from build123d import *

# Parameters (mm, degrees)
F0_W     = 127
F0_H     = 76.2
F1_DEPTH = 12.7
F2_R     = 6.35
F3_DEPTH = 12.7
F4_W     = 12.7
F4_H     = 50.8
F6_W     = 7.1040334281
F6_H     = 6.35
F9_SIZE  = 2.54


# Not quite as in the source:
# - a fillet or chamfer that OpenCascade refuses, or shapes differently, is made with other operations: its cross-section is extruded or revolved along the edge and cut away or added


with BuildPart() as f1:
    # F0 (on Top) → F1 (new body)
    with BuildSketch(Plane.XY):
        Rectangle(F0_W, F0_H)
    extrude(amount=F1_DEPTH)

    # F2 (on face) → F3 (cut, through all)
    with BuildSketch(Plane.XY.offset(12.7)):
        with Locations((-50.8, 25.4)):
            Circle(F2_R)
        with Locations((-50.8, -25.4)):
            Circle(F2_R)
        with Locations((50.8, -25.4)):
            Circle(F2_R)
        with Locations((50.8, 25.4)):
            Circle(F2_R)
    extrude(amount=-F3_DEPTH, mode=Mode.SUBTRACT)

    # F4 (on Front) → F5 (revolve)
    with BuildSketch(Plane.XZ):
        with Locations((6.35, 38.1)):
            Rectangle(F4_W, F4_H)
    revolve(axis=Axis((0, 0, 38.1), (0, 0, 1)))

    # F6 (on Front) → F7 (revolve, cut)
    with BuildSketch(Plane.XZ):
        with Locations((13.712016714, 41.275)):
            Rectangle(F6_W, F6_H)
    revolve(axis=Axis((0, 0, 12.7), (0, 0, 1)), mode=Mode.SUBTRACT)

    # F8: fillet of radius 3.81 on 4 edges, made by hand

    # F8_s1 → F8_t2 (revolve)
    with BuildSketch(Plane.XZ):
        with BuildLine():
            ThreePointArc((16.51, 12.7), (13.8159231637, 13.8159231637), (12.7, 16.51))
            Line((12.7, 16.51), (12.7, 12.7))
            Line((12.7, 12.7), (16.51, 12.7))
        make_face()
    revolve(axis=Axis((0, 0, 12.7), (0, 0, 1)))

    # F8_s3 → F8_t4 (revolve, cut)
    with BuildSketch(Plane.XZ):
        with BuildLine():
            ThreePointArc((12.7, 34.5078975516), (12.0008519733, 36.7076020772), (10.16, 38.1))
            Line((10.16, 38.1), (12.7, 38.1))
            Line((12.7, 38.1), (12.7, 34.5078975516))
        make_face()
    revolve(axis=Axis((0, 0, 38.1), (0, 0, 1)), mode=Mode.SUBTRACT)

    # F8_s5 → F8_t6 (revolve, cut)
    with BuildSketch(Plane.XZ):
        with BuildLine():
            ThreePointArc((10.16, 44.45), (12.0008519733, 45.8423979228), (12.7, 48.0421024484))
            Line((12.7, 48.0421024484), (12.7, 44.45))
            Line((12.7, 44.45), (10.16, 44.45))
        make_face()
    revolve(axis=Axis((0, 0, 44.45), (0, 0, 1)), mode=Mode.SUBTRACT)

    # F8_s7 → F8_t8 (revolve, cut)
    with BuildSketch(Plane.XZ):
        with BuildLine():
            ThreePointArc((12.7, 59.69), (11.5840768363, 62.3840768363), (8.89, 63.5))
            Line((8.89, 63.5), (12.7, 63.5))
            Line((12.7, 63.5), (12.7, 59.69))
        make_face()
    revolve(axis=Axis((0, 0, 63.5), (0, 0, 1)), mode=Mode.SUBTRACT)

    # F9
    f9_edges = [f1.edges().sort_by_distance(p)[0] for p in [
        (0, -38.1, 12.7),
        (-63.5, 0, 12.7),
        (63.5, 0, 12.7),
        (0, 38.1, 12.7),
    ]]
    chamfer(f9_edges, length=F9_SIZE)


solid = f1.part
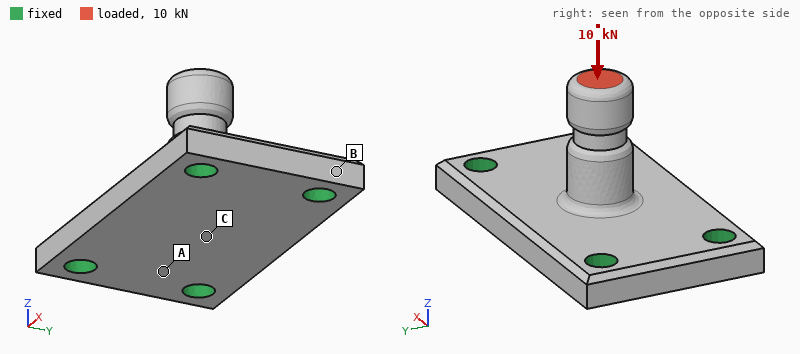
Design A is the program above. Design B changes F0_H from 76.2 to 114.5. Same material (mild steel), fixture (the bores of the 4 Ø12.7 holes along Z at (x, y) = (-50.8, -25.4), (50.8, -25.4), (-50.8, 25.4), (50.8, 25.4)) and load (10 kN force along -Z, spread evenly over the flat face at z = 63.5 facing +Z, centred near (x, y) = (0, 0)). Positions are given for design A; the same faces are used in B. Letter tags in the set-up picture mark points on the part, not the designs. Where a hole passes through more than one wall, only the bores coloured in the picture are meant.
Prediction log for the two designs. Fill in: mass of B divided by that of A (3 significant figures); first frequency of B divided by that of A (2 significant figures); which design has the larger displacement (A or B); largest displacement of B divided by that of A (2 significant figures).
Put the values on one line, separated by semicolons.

1.44; 1.0; A; 0.92
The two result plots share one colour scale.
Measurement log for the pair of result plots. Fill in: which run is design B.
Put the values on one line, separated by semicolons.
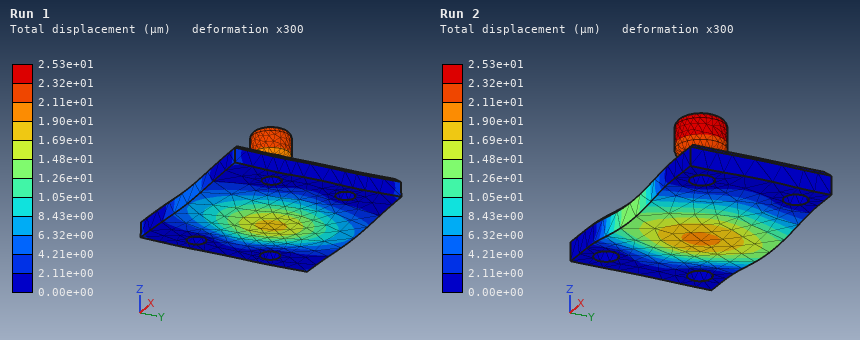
Run 1
